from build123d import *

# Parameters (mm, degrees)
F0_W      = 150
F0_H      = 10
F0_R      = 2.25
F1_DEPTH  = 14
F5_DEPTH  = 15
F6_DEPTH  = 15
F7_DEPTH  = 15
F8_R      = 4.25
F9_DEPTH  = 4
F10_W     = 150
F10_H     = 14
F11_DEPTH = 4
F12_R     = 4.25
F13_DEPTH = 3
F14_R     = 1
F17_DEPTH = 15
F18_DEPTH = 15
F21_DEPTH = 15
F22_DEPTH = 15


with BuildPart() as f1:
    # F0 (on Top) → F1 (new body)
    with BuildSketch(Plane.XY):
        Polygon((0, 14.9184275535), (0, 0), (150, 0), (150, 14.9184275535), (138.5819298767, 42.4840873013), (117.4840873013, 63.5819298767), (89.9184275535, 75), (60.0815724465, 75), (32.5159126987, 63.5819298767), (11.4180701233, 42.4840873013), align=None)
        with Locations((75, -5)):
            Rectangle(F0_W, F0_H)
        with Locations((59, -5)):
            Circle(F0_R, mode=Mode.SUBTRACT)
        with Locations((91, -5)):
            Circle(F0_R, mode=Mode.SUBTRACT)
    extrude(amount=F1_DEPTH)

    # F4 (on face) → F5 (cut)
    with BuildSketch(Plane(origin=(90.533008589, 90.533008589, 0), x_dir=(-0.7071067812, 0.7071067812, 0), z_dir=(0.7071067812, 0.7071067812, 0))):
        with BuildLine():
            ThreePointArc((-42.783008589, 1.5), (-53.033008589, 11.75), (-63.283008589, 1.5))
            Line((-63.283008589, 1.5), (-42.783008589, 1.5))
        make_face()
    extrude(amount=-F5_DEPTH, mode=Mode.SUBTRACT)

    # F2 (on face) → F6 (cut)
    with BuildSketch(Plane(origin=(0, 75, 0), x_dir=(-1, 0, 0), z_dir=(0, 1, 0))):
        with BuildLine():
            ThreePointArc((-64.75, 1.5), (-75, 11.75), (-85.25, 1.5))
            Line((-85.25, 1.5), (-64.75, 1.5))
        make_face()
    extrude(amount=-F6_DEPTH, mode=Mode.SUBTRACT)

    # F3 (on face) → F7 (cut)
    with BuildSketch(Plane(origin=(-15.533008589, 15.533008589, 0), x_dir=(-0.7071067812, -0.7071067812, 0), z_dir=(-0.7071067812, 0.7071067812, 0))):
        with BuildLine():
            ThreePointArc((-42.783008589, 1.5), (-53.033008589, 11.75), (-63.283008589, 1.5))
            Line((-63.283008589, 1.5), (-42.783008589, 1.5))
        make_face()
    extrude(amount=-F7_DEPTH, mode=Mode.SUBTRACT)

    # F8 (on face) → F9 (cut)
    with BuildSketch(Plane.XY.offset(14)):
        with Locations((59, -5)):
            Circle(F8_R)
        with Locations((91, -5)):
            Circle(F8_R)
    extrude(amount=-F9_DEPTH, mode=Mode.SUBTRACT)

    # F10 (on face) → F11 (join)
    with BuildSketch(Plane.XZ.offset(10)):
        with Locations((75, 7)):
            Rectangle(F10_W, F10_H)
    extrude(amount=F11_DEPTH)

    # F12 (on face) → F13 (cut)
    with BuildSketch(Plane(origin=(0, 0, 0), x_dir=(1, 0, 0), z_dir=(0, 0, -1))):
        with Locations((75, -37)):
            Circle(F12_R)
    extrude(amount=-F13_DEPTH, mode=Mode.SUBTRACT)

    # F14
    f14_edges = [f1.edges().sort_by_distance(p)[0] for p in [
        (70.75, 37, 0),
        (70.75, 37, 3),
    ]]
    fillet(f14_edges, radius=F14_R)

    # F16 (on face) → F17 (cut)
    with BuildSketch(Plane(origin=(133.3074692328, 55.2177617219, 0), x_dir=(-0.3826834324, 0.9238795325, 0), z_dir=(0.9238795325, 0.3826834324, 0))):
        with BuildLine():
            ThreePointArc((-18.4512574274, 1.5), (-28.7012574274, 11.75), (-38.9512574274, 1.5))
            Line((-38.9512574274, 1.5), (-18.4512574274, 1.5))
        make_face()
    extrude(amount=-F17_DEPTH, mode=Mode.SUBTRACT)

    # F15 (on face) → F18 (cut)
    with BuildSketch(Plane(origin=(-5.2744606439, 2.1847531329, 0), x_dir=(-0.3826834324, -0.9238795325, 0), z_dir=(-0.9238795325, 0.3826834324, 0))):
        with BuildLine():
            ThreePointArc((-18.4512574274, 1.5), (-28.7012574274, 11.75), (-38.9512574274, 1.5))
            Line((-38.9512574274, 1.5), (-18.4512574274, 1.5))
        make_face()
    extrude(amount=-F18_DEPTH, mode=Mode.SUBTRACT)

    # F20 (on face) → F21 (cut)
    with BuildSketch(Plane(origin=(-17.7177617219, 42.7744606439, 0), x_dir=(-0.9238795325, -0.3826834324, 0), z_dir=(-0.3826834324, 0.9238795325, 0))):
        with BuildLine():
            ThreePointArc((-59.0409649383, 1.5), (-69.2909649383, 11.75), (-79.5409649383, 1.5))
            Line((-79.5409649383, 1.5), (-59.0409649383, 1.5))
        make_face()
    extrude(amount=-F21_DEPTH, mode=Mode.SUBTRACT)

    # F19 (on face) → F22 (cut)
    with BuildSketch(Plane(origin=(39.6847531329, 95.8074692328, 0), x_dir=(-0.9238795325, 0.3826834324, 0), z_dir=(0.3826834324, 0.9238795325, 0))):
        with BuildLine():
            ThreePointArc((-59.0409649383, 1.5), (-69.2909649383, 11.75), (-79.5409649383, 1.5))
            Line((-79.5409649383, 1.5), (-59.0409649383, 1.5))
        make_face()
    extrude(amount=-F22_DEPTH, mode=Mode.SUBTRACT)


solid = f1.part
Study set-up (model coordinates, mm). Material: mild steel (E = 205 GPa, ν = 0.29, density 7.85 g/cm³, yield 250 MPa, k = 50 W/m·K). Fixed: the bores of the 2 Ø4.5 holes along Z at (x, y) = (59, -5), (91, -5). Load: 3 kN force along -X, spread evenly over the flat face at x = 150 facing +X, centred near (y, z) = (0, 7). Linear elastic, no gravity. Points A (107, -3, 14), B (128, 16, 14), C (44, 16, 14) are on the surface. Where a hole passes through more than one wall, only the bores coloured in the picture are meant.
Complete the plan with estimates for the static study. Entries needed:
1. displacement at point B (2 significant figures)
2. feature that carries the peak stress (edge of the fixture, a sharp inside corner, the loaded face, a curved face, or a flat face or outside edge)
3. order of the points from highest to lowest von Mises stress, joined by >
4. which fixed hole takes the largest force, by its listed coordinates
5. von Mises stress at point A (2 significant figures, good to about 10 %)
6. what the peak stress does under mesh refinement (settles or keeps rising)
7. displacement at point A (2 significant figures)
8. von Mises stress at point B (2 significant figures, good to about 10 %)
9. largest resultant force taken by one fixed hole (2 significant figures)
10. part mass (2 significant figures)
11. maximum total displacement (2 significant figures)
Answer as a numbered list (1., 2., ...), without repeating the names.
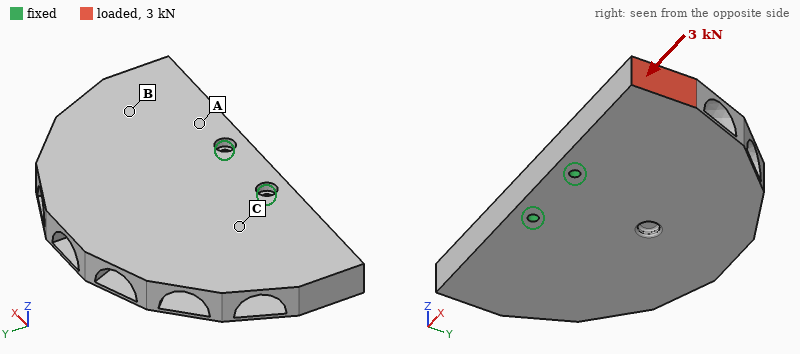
1. 1.7 µm
2. edge of the fixture
3. A > B > C
4. (91, -5)
5. 7.0 MPa
6. keeps rising
7. 1.2 µm
8. 3.9 MPa
9. 2.3 kN
10. 1.1 kg
11. 3.1 µm
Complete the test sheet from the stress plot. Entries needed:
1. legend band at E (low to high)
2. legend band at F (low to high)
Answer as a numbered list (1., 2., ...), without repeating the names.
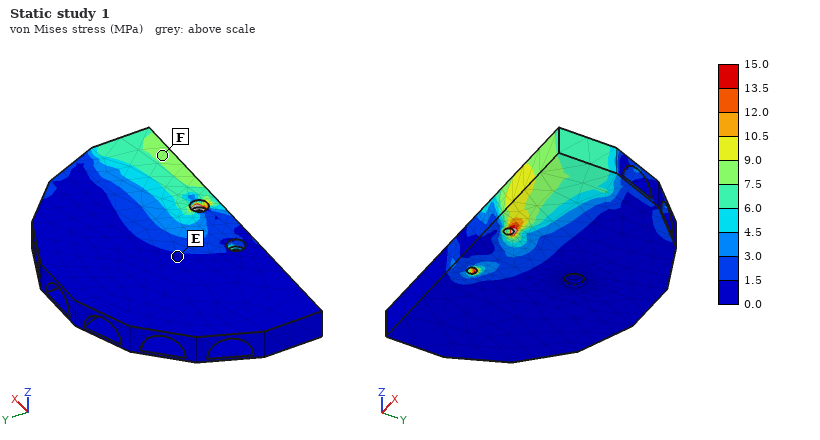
1. 0.0 to 1.5 MPa
2. 7.5 to 9.0 MPa
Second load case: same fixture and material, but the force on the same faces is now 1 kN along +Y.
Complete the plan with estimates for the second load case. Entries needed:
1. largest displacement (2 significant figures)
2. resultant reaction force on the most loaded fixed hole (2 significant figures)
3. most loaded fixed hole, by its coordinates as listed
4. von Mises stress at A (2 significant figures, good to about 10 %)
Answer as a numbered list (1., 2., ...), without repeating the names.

1. 8.4 µm
2. 2.7 kN
3. (91, -5)
4. 3.6 MPa
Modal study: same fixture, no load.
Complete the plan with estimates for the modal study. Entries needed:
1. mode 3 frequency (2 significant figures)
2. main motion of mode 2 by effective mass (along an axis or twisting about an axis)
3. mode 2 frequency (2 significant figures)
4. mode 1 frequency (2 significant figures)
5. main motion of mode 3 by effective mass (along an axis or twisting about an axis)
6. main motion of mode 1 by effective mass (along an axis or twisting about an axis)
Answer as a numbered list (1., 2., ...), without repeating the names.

1. 3000 Hz
2. twisting about Y
3. 2100 Hz
4. 1400 Hz
5. along Z
6. along Z
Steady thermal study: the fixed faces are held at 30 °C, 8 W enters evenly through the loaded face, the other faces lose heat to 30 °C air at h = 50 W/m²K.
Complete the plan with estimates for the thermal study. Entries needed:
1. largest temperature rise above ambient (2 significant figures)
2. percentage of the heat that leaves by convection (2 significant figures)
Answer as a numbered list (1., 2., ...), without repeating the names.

1. 15 K
2. 49 %
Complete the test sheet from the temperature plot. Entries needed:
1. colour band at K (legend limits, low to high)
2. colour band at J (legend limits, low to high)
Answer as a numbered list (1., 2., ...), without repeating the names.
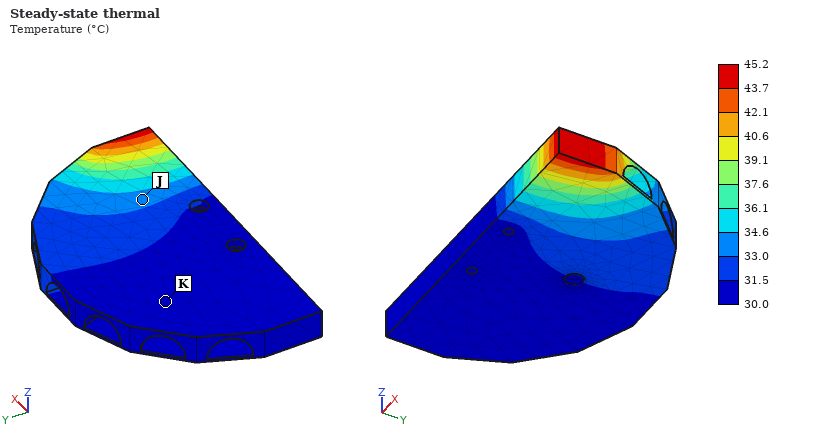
1. 30.0 to 31.5 °C
2. 33.0 to 34.6 °C
